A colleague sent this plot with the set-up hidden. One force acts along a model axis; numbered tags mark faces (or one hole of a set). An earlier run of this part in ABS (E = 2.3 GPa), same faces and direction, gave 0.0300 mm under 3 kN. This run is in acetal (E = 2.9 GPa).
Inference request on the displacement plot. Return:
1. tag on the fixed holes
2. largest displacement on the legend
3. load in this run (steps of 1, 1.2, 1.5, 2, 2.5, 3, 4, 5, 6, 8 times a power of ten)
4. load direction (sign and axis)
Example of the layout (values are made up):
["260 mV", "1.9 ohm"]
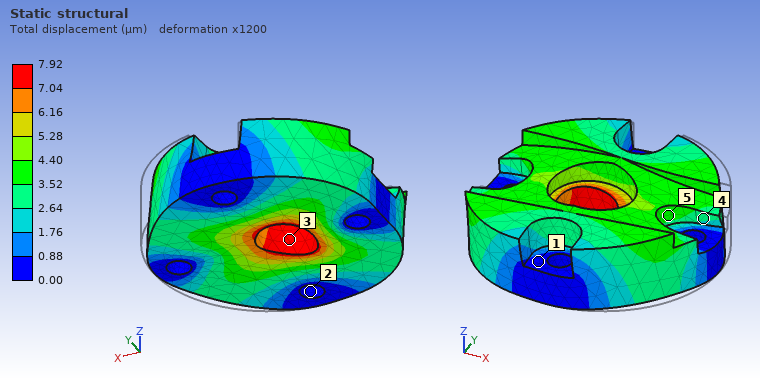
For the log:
["2", "7.92 µm", "1 kN", "-X"]
